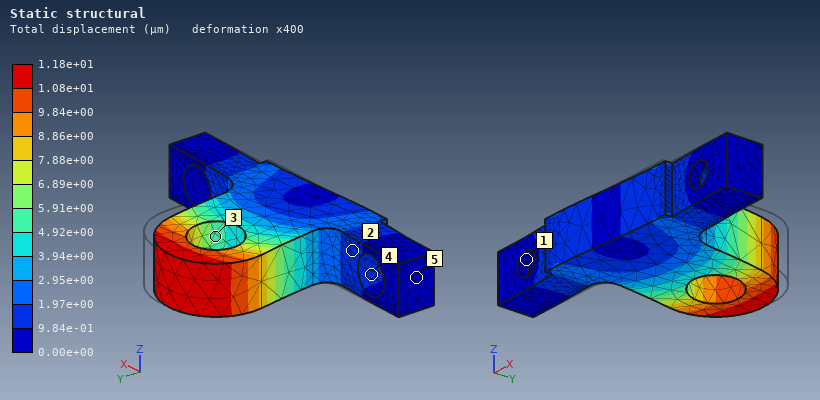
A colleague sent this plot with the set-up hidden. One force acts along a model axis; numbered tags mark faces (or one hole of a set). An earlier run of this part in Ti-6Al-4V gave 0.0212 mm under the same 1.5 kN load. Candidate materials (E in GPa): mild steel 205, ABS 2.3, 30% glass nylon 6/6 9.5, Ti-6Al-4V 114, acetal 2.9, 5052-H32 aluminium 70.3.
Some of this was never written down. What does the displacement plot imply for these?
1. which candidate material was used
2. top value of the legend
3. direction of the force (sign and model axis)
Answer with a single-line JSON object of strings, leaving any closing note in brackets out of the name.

{"which candidate material was used": "mild steel", "top value of the legend": "1.18e+01 µm", "direction of the force": "-X"}
